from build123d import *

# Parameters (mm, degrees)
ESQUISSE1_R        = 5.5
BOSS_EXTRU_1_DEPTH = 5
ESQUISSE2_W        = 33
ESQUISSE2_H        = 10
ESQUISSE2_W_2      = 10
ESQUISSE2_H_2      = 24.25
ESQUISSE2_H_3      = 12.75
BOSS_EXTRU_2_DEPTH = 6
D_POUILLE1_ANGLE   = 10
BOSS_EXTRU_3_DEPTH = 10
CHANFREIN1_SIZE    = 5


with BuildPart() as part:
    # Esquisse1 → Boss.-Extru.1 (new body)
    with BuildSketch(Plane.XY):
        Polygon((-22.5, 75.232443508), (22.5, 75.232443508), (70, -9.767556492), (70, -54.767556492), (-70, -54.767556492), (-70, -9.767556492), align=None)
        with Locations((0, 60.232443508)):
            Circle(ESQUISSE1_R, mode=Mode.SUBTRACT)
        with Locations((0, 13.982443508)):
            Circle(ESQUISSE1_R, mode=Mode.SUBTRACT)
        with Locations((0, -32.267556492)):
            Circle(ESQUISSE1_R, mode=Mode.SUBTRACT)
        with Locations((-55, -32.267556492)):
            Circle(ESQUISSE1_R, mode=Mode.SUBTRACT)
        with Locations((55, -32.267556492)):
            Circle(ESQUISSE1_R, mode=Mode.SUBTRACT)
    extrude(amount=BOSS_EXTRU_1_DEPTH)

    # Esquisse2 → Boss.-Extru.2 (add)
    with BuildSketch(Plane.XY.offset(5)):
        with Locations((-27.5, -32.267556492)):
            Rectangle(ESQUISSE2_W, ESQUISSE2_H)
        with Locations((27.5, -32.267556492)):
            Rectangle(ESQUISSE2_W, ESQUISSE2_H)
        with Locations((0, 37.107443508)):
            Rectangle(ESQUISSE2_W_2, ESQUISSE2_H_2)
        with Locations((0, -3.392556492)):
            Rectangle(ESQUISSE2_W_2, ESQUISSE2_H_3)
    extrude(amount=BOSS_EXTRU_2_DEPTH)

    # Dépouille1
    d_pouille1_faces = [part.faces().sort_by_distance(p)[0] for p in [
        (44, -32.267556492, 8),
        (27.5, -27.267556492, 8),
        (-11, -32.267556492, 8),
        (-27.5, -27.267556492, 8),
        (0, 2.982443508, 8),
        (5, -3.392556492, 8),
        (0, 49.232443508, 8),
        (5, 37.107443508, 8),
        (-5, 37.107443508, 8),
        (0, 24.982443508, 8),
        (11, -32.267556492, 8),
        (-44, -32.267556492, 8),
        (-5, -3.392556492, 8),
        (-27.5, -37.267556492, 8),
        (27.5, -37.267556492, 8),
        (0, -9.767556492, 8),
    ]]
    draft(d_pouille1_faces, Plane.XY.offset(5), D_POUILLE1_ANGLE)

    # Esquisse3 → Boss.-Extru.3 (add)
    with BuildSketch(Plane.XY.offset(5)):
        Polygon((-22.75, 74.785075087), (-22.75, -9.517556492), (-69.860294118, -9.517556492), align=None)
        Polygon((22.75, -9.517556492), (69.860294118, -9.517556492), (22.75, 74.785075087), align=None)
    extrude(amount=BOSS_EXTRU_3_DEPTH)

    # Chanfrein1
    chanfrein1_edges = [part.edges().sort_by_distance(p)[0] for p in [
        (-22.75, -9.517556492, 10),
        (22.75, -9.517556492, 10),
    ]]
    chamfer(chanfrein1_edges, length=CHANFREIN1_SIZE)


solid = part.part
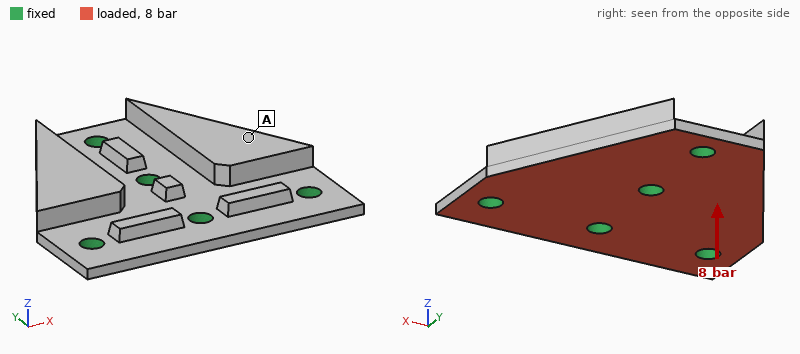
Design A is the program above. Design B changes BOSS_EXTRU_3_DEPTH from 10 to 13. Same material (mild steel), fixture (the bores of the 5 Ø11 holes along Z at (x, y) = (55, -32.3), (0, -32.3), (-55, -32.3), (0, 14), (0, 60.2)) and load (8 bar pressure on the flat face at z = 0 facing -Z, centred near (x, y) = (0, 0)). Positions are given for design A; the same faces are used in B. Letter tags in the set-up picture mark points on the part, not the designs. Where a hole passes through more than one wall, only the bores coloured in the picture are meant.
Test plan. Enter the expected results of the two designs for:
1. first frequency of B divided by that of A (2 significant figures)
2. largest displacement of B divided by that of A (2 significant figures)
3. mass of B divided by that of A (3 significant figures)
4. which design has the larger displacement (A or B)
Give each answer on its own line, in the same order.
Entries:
0.94
0.91
1.10
A
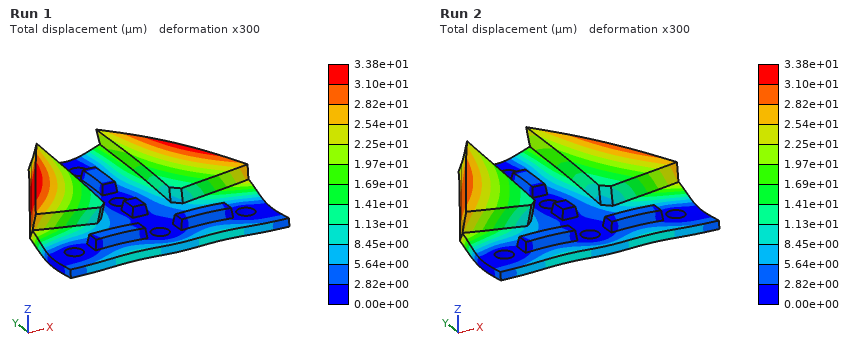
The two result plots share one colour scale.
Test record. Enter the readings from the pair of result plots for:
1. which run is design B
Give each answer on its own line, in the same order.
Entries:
Run 2
